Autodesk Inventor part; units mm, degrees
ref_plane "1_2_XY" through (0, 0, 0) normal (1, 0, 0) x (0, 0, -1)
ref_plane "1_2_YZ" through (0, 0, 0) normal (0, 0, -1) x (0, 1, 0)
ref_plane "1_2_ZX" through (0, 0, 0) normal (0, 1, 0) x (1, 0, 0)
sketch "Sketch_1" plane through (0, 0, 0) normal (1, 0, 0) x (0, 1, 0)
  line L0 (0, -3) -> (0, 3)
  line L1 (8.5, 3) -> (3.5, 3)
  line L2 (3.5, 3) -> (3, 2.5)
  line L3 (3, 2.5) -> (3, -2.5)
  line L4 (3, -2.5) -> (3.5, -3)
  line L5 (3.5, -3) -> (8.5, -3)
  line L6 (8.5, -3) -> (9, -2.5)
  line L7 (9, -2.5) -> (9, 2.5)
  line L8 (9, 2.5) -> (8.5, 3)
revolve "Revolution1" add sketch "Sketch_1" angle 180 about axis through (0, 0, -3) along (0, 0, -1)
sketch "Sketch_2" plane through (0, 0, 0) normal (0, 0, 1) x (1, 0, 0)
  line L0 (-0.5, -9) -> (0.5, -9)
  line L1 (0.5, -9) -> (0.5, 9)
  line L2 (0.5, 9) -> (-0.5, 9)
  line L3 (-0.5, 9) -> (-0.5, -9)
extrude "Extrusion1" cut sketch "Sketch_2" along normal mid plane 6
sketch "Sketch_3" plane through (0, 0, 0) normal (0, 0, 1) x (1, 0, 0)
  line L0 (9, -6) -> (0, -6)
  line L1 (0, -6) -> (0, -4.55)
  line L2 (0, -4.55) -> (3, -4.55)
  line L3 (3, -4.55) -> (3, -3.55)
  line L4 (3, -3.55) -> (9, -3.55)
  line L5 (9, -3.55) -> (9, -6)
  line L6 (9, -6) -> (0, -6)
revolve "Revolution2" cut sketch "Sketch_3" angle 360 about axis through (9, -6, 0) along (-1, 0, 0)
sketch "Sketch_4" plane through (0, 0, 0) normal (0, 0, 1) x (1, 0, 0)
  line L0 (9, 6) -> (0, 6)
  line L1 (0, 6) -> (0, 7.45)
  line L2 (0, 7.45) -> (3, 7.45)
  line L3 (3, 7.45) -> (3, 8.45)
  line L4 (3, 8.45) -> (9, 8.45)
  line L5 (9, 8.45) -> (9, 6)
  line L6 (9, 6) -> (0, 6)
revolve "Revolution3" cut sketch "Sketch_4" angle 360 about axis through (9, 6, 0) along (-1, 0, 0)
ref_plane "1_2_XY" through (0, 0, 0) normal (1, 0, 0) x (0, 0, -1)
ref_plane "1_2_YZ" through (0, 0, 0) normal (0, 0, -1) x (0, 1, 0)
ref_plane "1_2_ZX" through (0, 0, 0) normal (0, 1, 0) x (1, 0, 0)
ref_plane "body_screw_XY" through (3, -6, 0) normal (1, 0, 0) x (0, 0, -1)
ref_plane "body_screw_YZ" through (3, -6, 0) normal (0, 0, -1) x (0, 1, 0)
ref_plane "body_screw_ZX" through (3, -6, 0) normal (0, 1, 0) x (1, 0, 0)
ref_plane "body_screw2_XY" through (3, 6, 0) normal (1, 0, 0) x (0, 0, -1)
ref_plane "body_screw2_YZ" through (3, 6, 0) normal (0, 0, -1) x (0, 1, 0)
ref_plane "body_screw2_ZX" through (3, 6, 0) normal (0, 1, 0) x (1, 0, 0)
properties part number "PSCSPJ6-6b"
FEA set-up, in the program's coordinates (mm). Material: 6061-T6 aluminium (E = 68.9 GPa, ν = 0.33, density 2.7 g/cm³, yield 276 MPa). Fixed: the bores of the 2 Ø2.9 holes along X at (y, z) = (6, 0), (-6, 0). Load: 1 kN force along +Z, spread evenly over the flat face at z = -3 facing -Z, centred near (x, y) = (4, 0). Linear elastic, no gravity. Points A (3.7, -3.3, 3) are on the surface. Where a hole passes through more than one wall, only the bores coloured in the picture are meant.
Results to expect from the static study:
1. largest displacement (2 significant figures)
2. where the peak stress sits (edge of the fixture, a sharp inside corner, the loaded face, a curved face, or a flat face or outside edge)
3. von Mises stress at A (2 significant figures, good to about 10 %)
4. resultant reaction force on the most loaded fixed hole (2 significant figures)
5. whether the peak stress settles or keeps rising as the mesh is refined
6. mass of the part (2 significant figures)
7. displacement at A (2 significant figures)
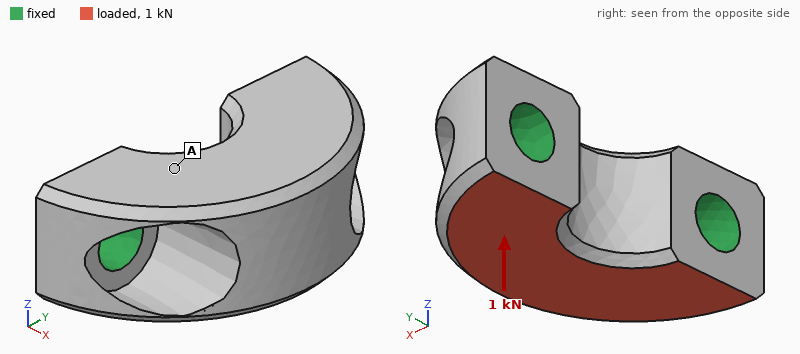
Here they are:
20 µm
edge of the fixture
29 MPa
500 N
keeps rising
1.3 g
8.5 µm
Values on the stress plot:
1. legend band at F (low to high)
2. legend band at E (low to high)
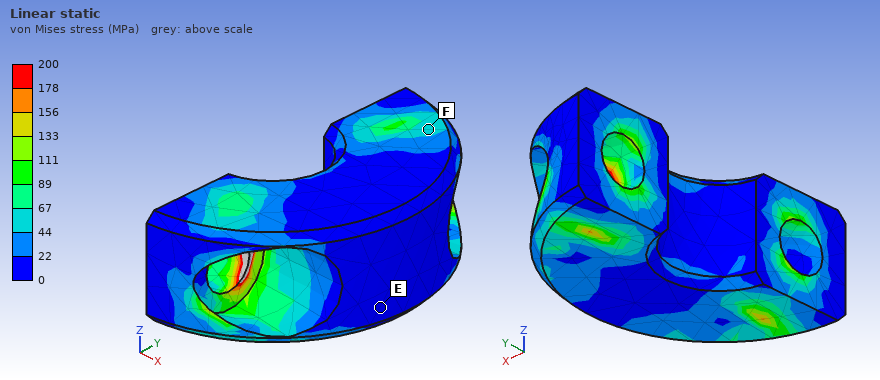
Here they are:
44 to 67 MPa
0 to 22 MPa
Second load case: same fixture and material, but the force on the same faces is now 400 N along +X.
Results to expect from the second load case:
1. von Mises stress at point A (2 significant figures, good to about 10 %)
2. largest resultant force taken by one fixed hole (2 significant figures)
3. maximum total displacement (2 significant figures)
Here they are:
10 MPa
210 N
6.8 µm
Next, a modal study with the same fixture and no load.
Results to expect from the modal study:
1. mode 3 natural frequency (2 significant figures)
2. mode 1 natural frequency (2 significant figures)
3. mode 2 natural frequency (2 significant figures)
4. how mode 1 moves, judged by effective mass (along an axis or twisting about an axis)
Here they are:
86 kHz
36 kHz
83 kHz
along Z
